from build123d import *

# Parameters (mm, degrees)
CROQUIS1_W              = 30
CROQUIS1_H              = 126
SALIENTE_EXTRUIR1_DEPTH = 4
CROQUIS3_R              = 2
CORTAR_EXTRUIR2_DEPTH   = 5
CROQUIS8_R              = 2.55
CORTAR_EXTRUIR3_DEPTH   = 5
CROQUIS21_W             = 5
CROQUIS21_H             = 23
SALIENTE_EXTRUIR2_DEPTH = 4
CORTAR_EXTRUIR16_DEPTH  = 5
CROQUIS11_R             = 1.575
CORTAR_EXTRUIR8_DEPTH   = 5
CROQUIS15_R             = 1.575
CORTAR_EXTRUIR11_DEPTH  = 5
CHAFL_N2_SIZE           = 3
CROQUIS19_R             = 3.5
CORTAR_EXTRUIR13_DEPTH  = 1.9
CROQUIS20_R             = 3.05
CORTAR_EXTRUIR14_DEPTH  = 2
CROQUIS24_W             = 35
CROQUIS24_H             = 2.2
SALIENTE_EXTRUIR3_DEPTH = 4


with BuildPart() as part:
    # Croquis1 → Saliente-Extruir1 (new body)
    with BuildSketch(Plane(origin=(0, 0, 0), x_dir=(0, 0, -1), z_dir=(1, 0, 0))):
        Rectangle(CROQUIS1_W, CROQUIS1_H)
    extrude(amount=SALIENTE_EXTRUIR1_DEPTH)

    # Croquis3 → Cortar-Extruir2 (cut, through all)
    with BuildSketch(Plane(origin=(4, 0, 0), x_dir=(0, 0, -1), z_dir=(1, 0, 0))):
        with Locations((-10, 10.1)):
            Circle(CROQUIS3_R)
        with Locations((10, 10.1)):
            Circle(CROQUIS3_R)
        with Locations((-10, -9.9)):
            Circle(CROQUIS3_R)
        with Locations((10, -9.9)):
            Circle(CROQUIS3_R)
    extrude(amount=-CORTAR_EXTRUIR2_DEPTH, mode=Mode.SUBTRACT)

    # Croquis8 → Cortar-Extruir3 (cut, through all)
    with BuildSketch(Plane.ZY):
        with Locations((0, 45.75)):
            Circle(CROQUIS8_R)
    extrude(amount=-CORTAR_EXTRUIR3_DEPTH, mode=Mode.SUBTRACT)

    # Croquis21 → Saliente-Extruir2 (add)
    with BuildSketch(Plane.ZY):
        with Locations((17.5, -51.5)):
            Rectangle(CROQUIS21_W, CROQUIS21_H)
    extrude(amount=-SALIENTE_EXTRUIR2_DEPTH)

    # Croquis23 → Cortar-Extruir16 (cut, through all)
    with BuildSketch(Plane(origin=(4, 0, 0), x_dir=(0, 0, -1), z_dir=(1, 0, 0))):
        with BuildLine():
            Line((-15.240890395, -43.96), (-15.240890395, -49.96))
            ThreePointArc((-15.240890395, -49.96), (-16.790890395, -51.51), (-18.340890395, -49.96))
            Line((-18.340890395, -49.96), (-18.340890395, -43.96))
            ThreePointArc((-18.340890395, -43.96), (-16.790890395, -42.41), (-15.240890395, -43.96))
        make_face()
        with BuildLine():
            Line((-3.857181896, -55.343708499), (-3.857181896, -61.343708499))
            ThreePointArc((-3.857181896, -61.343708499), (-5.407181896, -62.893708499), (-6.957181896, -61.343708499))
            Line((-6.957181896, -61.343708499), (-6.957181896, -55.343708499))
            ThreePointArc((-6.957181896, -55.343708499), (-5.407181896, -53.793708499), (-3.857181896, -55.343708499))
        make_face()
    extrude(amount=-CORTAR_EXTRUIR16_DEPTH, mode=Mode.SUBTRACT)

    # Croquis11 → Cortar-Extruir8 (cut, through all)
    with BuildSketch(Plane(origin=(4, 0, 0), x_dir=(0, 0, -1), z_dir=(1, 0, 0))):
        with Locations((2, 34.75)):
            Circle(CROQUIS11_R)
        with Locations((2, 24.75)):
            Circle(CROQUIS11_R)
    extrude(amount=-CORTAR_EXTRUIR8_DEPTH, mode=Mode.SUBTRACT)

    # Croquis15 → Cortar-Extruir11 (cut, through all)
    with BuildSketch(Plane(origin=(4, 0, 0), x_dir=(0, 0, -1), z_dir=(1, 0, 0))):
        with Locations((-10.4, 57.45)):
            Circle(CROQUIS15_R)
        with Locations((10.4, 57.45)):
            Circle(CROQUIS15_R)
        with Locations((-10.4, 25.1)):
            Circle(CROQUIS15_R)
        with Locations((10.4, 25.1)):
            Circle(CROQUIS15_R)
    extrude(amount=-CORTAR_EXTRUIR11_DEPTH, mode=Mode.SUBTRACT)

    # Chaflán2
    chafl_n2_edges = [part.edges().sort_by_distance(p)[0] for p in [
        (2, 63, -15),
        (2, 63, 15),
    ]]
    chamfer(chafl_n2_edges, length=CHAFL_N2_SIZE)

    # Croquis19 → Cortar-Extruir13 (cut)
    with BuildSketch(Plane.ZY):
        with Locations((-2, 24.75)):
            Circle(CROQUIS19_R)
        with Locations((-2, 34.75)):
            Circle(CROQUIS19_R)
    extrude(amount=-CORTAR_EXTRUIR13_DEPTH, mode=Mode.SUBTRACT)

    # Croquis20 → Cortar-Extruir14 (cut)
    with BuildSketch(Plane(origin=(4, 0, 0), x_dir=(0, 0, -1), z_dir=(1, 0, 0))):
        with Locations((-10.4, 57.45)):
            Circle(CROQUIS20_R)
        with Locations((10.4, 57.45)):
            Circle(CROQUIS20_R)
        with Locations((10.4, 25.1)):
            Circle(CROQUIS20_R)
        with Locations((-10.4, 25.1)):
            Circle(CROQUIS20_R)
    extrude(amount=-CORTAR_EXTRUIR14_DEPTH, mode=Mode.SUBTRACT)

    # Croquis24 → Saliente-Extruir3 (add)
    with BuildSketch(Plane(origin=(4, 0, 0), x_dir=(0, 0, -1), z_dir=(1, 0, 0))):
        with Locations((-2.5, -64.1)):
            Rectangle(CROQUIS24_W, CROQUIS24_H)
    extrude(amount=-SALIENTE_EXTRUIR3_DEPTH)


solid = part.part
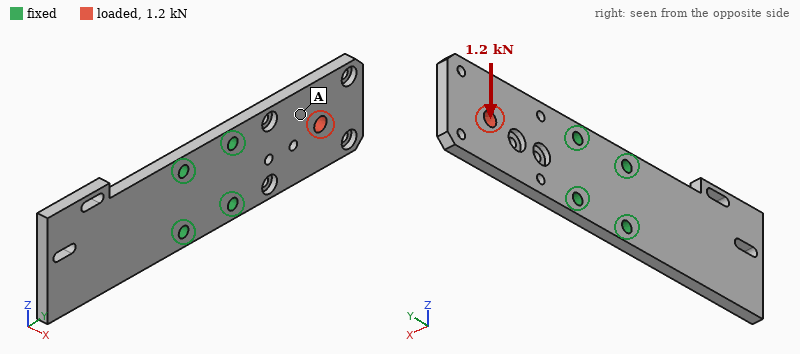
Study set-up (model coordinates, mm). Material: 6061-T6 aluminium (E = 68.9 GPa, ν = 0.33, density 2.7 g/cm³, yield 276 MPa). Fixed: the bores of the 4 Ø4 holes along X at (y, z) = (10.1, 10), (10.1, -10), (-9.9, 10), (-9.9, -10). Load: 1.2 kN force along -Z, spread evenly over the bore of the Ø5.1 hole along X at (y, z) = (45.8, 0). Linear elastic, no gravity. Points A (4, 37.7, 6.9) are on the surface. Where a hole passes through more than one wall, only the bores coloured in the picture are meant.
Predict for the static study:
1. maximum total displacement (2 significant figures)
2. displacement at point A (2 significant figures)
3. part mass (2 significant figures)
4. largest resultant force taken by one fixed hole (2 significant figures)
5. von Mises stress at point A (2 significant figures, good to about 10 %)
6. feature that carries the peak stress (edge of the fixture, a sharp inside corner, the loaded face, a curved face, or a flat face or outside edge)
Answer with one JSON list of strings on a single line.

["86 µm", "41 µm", "40 g", "1.9 kN", "17 MPa", "a curved face"]
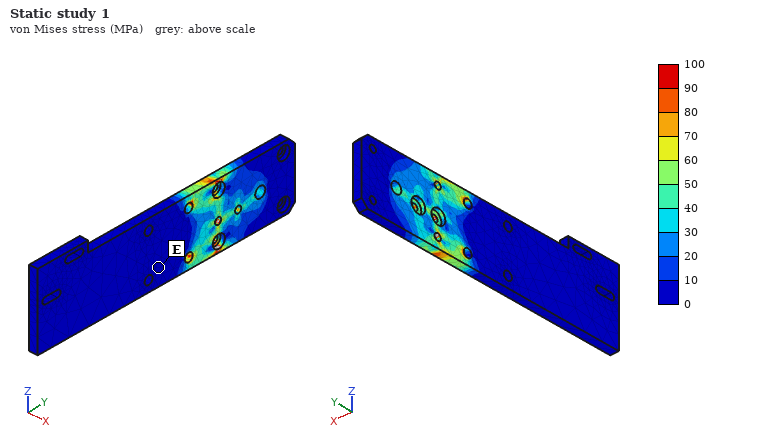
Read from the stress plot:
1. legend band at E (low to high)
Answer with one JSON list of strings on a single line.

["0 to 10 MPa"]
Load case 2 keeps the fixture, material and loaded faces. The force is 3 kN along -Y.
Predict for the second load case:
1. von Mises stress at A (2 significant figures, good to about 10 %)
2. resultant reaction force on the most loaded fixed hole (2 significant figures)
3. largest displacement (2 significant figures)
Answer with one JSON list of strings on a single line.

["25 MPa", "1.4 kN", "22 µm"]
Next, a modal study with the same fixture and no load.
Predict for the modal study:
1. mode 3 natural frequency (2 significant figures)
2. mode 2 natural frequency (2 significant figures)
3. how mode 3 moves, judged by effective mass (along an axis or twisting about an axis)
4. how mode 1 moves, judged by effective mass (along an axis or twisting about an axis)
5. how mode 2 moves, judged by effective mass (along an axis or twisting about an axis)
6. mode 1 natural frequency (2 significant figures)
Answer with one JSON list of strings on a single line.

["3500 Hz", "1200 Hz", "twisting about Y", "along X", "along X", "1000 Hz"]
